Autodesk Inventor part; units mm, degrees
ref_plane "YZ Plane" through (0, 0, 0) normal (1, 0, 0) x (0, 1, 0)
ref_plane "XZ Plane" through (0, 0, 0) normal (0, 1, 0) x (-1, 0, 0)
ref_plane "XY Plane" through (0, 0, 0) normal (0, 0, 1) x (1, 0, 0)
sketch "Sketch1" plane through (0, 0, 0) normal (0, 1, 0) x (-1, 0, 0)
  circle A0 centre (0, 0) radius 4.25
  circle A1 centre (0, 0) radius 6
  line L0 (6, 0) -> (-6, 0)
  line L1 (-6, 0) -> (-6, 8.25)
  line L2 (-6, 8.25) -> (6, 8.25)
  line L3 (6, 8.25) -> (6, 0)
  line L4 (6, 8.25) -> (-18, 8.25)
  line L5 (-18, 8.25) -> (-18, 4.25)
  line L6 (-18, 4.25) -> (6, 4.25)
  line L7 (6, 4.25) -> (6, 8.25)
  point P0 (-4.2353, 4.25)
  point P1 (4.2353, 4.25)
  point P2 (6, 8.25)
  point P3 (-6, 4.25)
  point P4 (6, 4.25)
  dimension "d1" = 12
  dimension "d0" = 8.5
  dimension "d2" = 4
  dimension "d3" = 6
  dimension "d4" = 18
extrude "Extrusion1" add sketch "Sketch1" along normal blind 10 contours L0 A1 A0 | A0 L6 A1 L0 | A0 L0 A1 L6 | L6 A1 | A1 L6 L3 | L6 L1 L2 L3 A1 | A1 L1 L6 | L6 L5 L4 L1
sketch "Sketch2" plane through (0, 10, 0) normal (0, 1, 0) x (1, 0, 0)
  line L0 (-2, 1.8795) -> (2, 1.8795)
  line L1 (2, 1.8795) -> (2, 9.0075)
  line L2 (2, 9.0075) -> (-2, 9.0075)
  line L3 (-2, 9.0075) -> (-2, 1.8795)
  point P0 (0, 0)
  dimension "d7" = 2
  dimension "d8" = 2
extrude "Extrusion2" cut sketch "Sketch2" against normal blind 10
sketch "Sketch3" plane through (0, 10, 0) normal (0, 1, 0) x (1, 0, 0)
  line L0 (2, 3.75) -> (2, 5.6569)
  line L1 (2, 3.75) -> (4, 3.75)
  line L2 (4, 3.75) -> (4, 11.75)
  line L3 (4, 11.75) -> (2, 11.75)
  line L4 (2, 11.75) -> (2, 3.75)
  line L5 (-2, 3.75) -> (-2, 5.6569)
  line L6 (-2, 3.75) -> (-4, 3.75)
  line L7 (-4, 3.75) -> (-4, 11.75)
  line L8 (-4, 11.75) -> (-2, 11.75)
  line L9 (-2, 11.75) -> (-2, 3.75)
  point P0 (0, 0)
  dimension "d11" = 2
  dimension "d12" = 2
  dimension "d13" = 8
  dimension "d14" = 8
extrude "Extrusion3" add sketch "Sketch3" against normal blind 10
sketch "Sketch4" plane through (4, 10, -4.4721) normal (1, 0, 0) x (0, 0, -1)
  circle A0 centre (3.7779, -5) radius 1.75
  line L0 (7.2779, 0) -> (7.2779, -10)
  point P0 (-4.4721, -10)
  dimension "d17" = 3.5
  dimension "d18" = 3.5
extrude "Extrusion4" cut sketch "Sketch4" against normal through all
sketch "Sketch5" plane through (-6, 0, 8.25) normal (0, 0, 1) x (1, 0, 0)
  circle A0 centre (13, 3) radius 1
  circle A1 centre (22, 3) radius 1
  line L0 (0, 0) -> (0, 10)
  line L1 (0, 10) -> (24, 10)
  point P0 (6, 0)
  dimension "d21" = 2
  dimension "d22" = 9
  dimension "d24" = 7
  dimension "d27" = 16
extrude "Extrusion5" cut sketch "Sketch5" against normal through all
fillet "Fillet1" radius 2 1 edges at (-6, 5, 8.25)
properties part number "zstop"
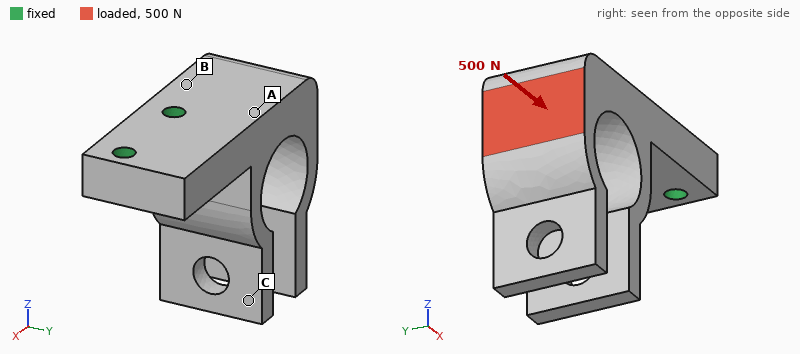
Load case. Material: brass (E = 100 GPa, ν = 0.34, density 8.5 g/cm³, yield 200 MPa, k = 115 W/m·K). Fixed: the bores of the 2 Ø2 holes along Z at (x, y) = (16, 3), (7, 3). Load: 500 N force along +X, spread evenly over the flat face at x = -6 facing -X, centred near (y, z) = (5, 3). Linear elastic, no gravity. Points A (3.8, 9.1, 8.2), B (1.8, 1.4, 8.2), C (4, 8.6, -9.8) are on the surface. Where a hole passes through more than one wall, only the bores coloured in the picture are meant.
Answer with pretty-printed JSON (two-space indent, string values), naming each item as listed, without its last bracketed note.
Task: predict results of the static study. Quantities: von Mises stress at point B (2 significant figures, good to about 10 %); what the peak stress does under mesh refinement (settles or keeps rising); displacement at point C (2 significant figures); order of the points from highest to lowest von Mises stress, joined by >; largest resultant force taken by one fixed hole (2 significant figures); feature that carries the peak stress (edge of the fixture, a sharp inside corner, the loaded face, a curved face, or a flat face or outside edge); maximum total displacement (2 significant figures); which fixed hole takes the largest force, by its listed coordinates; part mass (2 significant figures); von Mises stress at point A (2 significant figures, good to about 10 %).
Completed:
{
  "von Mises stress at point B": "38 MPa",
  "what the peak stress does under mesh refinement": "keeps rising",
  "displacement at point C": "16 µm",
  "order of the points from highest to lowest von Mises stress, joined by >": "B > A > C",
  "largest resultant force taken by one fixed hole": "410 N",
  "feature that carries the peak stress": "edge of the fixture",
  "maximum total displacement": "59 µm",
  "which fixed hole takes the largest force, by its listed coordinates": "(7, 3)",
  "part mass": "13 g",
  "von Mises stress at point A": "21 MPa"
}
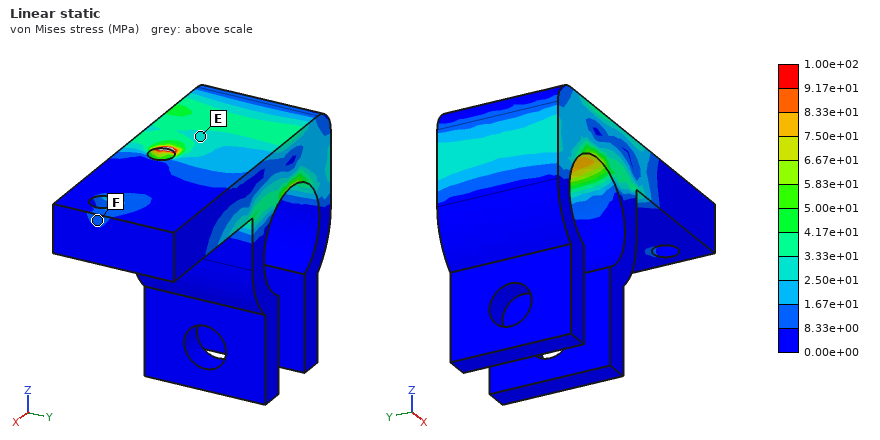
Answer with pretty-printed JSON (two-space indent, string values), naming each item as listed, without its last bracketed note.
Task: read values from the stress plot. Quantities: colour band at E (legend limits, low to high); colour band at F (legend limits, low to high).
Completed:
{
  "colour band at E": "2.50e+01 to 3.33e+01 MPa",
  "colour band at F": "8.33e+00 to 1.67e+01 MPa"
}
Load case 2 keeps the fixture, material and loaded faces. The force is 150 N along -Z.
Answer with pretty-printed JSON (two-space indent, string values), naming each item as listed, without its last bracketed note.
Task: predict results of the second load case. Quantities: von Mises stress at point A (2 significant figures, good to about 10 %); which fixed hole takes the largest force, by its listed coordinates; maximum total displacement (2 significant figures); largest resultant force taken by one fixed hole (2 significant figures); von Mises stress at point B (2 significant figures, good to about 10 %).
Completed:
{
  "von Mises stress at point A": "30 MPa",
  "which fixed hole takes the largest force, by its listed coordinates": "(7, 3)",
  "maximum total displacement": "44 µm",
  "largest resultant force taken by one fixed hole": "210 N",
  "von Mises stress at point B": "38 MPa"
}
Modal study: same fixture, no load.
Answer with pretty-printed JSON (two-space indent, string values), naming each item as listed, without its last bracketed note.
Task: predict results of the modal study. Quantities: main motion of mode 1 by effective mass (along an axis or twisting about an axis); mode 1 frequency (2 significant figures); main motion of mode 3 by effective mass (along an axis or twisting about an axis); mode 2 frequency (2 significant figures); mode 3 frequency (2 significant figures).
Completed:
{
  "main motion of mode 1 by effective mass": "along X",
  "mode 1 frequency": "3800 Hz",
  "main motion of mode 3 by effective mass": "along Y",
  "mode 2 frequency": "4500 Hz",
  "mode 3 frequency": "5900 Hz"
}
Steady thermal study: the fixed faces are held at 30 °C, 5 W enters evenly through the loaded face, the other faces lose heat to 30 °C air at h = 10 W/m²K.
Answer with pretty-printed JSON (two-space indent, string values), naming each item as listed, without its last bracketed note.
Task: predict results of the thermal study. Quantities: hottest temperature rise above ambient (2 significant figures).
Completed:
{
  "hottest temperature rise above ambient": "15 K"
}
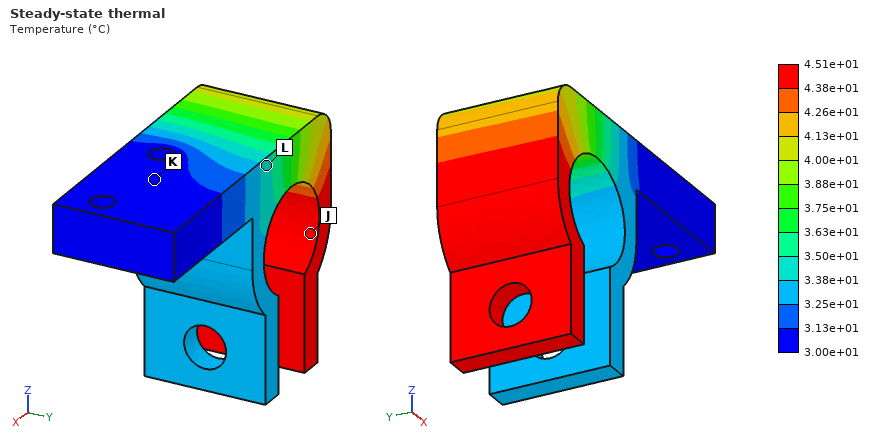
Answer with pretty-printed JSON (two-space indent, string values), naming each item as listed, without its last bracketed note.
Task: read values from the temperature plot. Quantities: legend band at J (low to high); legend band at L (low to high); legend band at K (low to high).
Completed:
{
  "legend band at J": "4.38e+01 to 4.51e+01 °C",
  "legend band at L": "3.38e+01 to 3.50e+01 °C",
  "legend band at K": "3.00e+01 to 3.13e+01 °C"
}
